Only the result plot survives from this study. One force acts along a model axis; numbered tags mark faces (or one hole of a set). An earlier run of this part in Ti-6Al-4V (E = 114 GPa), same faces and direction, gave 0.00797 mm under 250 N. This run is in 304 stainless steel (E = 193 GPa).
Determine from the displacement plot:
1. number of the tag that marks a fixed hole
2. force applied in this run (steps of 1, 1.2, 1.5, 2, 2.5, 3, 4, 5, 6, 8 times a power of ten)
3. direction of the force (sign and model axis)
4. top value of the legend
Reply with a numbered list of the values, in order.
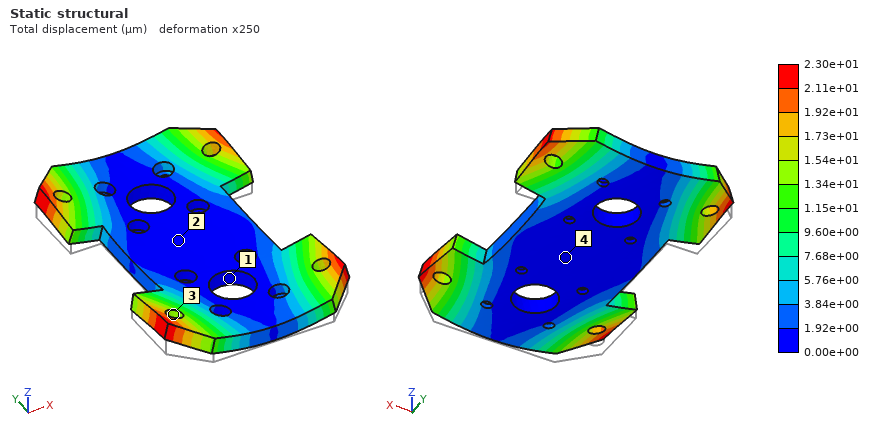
1. 1
2. 1.2 kN
3. +Z
4. 2.30e+01 µm
